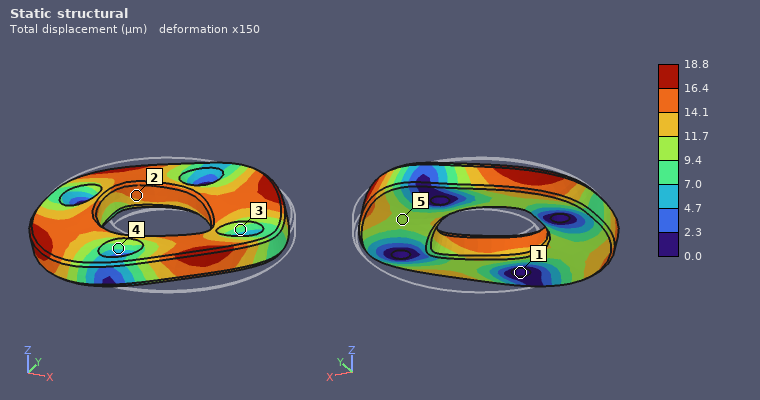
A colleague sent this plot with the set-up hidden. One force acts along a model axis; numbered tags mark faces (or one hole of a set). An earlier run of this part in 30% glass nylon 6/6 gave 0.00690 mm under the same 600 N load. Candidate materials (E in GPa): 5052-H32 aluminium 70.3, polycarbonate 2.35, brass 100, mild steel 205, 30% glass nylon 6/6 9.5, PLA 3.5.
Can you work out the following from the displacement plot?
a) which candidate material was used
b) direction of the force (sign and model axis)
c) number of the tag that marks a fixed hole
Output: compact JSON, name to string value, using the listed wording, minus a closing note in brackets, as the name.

{"which candidate material was used": "PLA", "direction of the force": "-X", "number of the tag that marks a fixed hole": "1"}
